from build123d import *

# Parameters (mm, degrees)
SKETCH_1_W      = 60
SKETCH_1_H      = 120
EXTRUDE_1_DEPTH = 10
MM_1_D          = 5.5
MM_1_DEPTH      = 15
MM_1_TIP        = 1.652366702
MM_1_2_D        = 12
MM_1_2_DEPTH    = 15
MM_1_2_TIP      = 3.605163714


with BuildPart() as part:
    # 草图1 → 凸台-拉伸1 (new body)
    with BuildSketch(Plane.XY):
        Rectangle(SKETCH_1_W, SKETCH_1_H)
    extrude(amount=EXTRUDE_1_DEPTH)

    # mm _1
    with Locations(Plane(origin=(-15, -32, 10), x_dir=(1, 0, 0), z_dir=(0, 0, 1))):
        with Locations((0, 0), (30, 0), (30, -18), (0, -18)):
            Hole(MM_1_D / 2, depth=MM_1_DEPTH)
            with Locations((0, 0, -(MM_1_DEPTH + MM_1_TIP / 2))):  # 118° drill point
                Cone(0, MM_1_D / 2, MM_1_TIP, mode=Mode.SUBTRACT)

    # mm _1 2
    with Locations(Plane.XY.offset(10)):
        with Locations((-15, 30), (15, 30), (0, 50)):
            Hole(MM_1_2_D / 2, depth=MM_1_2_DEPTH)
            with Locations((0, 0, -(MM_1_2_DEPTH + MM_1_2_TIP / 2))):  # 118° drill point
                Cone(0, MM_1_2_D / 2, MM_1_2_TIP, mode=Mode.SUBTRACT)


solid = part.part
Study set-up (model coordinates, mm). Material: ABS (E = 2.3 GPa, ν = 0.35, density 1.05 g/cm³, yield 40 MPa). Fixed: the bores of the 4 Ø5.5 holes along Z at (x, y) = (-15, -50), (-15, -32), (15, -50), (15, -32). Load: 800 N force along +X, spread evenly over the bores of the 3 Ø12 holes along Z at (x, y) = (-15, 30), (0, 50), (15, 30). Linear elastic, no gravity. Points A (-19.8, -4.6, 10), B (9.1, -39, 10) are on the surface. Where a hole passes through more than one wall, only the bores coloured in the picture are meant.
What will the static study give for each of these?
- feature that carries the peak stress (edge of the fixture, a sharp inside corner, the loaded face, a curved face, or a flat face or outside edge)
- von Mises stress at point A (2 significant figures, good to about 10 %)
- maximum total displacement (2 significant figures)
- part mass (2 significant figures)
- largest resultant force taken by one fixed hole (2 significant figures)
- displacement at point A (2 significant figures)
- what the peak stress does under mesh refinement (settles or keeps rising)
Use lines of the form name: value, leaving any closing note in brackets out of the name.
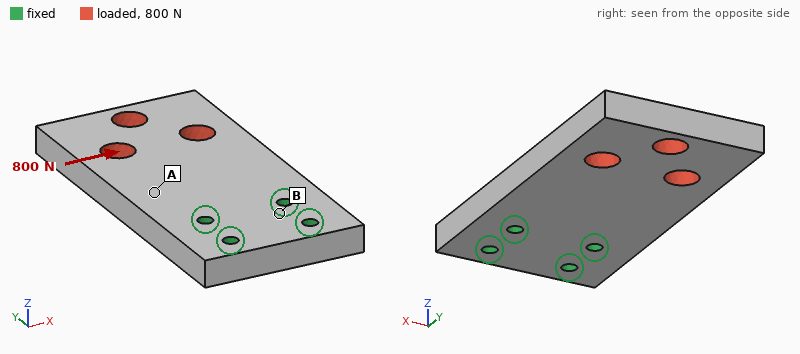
feature that carries the peak stress: edge of the fixture
von Mises stress at point A: 4.1 MPa
maximum total displacement: 0.60 mm
part mass: 71 g
largest resultant force taken by one fixed hole: 1.3 kN
displacement at point A: 0.15 mm
what the peak stress does under mesh refinement: keeps rising
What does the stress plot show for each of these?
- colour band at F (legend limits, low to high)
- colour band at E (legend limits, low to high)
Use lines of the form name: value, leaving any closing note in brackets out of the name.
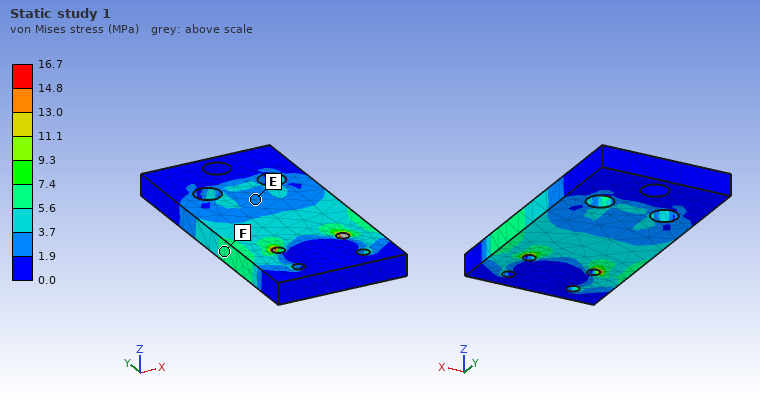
colour band at F: 5.6 to 7.4 MPa
colour band at E: 1.9 to 3.7 MPa
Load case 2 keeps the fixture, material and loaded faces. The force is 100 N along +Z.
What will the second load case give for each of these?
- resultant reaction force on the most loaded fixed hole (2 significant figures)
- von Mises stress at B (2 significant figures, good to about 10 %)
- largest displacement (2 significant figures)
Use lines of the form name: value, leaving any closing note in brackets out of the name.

resultant reaction force on the most loaded fixed hole: 110 N
von Mises stress at B: 1.3 MPa
largest displacement: 1.5 mm
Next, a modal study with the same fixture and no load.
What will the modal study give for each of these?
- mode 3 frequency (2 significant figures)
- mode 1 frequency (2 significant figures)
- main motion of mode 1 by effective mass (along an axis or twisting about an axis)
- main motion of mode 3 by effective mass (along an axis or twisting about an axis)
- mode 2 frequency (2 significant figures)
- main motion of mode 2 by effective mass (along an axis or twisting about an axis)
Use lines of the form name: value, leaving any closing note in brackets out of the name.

mode 3 frequency: 1200 Hz
mode 1 frequency: 290 Hz
main motion of mode 1 by effective mass: along Z
main motion of mode 3 by effective mass: along X
mode 2 frequency: 860 Hz
main motion of mode 2 by effective mass: twisting about Y
